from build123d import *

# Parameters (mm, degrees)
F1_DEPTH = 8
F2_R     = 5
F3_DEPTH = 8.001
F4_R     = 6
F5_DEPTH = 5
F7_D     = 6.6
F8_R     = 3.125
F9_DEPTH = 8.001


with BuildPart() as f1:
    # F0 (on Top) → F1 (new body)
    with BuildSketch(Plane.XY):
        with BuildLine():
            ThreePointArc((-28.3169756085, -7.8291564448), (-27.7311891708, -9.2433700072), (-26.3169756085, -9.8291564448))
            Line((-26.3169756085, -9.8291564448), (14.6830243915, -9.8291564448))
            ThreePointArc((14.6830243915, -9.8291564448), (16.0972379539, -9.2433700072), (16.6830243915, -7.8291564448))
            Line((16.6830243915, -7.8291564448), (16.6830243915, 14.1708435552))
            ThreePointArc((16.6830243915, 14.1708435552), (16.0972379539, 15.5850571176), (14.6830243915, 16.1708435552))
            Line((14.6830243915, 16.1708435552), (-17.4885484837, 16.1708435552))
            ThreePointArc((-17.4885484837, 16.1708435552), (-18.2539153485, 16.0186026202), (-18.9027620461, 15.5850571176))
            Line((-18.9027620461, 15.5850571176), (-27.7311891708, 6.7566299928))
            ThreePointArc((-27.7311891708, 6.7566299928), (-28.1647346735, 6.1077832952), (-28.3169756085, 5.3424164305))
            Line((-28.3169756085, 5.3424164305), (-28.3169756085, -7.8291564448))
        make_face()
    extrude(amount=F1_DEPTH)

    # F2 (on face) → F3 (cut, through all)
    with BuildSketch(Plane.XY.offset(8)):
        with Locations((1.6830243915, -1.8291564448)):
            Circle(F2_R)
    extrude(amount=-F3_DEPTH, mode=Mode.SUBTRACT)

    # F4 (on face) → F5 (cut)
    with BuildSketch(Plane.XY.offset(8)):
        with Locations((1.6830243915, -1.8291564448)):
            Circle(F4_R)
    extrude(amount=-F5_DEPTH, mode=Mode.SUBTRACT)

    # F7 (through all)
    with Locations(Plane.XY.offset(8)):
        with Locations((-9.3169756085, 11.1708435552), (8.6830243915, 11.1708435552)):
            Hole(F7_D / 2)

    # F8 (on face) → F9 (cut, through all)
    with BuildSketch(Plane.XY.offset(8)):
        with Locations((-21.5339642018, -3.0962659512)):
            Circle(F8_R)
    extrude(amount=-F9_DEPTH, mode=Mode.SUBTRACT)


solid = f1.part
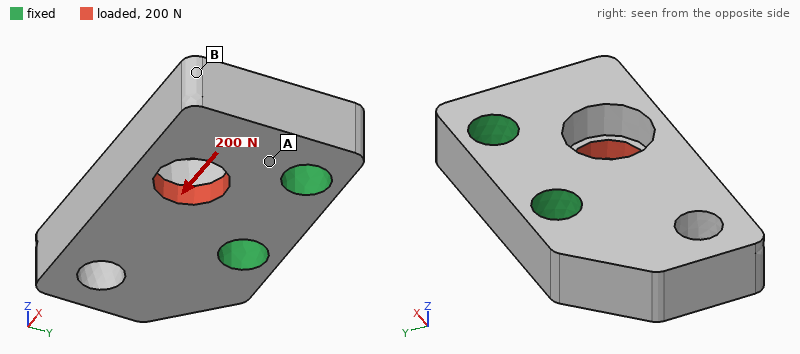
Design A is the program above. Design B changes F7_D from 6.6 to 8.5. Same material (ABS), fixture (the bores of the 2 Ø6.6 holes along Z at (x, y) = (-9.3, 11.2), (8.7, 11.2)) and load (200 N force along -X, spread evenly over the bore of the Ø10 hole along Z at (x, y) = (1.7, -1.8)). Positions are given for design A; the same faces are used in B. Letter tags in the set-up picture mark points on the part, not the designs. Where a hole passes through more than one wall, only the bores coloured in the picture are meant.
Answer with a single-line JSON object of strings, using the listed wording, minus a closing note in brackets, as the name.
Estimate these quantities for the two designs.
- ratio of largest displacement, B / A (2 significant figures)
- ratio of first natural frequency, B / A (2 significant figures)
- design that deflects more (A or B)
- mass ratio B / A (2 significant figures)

{"ratio of largest displacement, B / A": "0.86", "ratio of first natural frequency, B / A": "1.1", "design that deflects more": "A", "mass ratio B / A": "0.95"}
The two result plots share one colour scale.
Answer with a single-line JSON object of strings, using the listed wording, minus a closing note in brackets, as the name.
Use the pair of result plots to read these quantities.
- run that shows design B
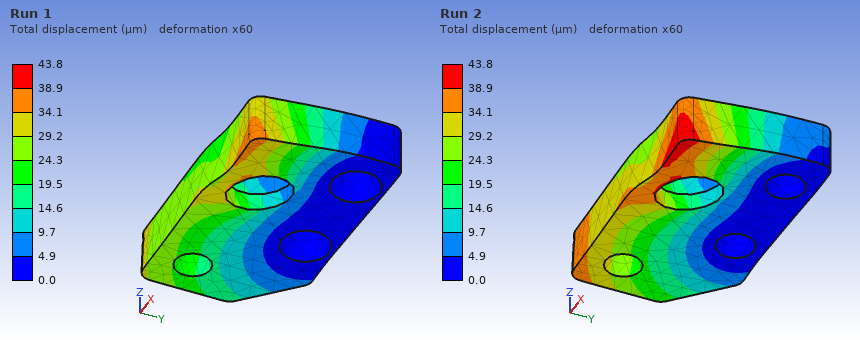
{"run that shows design B": "Run 1"}
